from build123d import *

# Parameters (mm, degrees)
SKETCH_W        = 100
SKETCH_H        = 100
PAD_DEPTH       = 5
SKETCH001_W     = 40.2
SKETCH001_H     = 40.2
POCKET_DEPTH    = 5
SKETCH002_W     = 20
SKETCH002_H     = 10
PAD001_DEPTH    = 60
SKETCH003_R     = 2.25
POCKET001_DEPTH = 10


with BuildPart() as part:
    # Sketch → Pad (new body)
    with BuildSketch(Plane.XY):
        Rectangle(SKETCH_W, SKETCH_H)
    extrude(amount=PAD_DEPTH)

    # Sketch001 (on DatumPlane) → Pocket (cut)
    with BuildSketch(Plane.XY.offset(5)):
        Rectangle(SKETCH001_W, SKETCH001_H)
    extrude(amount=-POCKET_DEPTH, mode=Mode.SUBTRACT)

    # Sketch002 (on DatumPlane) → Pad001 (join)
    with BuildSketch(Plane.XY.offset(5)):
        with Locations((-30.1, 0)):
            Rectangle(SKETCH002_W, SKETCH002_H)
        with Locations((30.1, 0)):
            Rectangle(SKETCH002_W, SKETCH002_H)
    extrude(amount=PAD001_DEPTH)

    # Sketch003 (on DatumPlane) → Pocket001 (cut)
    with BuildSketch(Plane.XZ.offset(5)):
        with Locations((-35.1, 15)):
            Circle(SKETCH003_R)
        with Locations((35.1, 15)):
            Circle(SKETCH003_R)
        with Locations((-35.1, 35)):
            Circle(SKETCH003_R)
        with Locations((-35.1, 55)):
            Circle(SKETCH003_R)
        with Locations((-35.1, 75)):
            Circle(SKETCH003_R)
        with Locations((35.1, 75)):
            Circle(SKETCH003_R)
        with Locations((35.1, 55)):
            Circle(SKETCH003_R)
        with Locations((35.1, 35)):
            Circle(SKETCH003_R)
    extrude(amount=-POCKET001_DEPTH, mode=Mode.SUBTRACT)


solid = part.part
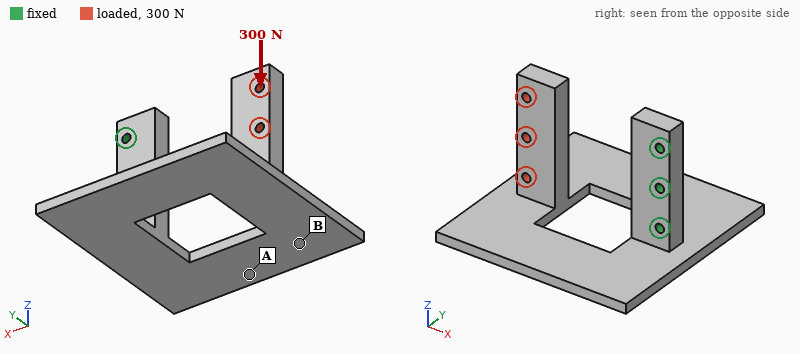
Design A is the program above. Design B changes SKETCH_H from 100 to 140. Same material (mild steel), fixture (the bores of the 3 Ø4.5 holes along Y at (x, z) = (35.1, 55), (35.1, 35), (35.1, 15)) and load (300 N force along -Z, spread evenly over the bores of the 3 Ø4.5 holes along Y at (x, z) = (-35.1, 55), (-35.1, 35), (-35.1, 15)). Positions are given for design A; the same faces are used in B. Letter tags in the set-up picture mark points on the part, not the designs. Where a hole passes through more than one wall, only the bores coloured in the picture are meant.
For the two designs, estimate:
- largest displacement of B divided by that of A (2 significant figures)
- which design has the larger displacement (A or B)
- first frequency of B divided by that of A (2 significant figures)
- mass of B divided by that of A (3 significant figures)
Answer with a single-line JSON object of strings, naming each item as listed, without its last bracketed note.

{"largest displacement of B divided by that of A": "0.84", "which design has the larger displacement": "A", "first frequency of B divided by that of A": "0.96", "mass of B divided by that of A": "1.31"}
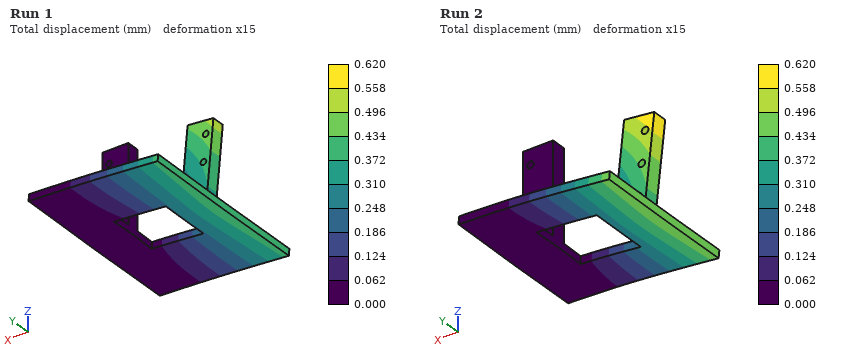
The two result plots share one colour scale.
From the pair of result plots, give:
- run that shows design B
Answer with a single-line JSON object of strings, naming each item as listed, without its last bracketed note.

{"run that shows design B": "Run 1"}
